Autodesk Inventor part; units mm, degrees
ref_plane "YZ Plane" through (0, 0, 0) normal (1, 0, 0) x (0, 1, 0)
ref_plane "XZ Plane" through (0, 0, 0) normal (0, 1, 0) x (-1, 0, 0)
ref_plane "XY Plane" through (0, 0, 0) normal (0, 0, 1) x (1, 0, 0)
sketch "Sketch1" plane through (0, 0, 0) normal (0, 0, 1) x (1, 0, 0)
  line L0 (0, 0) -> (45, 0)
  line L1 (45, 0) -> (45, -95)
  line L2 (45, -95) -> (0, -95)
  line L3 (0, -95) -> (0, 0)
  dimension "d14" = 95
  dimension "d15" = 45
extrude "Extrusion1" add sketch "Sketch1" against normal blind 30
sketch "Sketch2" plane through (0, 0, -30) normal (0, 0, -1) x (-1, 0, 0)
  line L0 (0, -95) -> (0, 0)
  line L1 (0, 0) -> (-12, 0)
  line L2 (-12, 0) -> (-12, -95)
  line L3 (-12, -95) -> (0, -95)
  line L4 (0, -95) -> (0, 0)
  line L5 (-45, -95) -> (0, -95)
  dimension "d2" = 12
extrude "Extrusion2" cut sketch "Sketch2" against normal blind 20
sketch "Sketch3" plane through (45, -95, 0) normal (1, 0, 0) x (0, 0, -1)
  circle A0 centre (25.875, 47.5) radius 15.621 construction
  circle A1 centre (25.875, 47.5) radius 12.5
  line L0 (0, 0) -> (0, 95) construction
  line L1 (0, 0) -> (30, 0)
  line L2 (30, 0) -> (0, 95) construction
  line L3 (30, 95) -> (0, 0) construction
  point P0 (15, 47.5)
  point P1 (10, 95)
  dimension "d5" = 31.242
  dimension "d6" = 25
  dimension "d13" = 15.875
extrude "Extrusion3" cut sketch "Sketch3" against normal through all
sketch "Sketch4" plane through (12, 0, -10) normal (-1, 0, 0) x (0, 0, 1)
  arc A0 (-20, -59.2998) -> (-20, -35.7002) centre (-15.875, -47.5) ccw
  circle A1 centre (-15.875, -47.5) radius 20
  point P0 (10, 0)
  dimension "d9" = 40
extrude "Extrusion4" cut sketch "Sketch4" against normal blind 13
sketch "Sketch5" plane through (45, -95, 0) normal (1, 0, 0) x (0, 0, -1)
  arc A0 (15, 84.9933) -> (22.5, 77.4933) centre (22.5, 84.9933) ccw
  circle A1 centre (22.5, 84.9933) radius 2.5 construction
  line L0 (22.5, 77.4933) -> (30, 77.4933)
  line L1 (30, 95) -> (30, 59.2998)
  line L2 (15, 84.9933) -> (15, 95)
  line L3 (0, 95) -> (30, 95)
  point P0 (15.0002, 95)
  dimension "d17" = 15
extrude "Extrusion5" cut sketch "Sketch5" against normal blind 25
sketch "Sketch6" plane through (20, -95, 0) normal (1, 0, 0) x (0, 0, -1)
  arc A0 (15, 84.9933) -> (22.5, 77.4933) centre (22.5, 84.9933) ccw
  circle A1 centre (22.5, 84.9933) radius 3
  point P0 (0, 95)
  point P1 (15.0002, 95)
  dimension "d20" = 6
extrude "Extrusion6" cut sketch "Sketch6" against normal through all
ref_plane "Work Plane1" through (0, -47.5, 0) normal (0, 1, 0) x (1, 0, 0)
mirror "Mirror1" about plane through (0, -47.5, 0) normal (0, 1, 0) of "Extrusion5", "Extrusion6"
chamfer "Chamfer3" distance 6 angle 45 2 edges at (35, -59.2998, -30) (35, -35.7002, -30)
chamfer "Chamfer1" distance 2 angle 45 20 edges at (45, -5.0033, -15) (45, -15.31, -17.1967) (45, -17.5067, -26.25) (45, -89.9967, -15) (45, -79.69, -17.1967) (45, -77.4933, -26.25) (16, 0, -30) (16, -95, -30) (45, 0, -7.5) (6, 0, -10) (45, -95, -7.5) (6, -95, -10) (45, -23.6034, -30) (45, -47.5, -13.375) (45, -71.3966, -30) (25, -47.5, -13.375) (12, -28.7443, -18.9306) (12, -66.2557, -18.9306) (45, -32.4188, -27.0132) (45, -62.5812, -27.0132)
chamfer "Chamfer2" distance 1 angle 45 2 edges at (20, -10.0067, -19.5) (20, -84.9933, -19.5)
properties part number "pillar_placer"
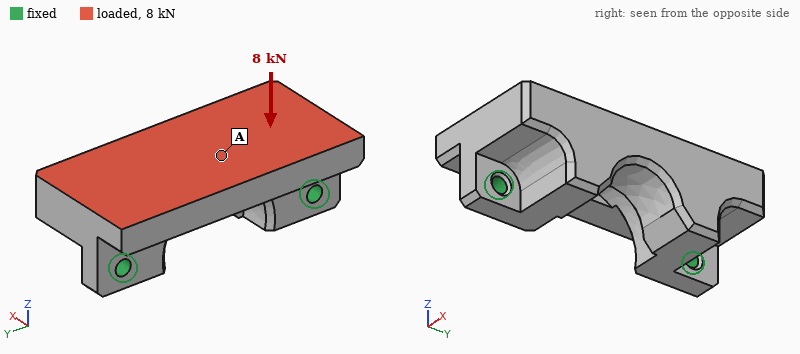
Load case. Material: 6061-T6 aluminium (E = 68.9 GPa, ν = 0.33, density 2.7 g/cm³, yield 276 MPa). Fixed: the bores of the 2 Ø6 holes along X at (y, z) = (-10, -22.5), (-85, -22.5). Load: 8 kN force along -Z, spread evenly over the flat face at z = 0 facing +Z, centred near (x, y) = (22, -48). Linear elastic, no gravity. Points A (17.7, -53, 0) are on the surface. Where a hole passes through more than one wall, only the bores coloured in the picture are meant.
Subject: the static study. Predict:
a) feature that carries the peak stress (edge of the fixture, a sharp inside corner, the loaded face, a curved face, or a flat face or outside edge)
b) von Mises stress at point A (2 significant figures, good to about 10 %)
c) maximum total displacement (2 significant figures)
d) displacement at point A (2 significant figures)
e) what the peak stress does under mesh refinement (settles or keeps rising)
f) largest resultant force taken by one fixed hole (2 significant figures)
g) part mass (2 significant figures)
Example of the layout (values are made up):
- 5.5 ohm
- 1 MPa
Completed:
- edge of the fixture
- 17 MPa
- 98 µm
- 52 µm
- keeps rising
- 4.5 kN
- 200 g
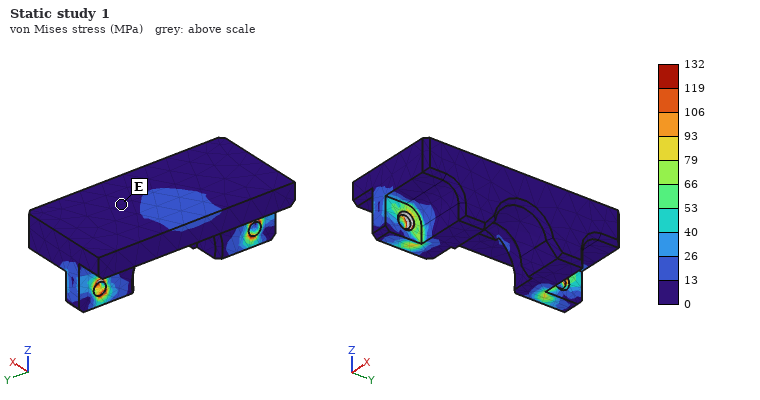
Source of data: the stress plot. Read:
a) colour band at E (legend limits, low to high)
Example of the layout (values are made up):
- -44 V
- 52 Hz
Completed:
- 0 to 13 MPa
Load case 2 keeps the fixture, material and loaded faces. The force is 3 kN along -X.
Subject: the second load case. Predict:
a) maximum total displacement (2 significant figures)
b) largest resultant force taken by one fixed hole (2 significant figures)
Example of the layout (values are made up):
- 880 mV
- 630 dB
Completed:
- 0.10 mm
- 1.5 kN
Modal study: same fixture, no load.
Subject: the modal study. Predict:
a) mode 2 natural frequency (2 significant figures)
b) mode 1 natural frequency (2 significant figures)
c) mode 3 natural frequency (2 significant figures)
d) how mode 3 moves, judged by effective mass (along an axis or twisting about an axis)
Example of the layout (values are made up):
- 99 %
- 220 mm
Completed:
- 6300 Hz
- 2600 Hz
- 9400 Hz
- along Y
